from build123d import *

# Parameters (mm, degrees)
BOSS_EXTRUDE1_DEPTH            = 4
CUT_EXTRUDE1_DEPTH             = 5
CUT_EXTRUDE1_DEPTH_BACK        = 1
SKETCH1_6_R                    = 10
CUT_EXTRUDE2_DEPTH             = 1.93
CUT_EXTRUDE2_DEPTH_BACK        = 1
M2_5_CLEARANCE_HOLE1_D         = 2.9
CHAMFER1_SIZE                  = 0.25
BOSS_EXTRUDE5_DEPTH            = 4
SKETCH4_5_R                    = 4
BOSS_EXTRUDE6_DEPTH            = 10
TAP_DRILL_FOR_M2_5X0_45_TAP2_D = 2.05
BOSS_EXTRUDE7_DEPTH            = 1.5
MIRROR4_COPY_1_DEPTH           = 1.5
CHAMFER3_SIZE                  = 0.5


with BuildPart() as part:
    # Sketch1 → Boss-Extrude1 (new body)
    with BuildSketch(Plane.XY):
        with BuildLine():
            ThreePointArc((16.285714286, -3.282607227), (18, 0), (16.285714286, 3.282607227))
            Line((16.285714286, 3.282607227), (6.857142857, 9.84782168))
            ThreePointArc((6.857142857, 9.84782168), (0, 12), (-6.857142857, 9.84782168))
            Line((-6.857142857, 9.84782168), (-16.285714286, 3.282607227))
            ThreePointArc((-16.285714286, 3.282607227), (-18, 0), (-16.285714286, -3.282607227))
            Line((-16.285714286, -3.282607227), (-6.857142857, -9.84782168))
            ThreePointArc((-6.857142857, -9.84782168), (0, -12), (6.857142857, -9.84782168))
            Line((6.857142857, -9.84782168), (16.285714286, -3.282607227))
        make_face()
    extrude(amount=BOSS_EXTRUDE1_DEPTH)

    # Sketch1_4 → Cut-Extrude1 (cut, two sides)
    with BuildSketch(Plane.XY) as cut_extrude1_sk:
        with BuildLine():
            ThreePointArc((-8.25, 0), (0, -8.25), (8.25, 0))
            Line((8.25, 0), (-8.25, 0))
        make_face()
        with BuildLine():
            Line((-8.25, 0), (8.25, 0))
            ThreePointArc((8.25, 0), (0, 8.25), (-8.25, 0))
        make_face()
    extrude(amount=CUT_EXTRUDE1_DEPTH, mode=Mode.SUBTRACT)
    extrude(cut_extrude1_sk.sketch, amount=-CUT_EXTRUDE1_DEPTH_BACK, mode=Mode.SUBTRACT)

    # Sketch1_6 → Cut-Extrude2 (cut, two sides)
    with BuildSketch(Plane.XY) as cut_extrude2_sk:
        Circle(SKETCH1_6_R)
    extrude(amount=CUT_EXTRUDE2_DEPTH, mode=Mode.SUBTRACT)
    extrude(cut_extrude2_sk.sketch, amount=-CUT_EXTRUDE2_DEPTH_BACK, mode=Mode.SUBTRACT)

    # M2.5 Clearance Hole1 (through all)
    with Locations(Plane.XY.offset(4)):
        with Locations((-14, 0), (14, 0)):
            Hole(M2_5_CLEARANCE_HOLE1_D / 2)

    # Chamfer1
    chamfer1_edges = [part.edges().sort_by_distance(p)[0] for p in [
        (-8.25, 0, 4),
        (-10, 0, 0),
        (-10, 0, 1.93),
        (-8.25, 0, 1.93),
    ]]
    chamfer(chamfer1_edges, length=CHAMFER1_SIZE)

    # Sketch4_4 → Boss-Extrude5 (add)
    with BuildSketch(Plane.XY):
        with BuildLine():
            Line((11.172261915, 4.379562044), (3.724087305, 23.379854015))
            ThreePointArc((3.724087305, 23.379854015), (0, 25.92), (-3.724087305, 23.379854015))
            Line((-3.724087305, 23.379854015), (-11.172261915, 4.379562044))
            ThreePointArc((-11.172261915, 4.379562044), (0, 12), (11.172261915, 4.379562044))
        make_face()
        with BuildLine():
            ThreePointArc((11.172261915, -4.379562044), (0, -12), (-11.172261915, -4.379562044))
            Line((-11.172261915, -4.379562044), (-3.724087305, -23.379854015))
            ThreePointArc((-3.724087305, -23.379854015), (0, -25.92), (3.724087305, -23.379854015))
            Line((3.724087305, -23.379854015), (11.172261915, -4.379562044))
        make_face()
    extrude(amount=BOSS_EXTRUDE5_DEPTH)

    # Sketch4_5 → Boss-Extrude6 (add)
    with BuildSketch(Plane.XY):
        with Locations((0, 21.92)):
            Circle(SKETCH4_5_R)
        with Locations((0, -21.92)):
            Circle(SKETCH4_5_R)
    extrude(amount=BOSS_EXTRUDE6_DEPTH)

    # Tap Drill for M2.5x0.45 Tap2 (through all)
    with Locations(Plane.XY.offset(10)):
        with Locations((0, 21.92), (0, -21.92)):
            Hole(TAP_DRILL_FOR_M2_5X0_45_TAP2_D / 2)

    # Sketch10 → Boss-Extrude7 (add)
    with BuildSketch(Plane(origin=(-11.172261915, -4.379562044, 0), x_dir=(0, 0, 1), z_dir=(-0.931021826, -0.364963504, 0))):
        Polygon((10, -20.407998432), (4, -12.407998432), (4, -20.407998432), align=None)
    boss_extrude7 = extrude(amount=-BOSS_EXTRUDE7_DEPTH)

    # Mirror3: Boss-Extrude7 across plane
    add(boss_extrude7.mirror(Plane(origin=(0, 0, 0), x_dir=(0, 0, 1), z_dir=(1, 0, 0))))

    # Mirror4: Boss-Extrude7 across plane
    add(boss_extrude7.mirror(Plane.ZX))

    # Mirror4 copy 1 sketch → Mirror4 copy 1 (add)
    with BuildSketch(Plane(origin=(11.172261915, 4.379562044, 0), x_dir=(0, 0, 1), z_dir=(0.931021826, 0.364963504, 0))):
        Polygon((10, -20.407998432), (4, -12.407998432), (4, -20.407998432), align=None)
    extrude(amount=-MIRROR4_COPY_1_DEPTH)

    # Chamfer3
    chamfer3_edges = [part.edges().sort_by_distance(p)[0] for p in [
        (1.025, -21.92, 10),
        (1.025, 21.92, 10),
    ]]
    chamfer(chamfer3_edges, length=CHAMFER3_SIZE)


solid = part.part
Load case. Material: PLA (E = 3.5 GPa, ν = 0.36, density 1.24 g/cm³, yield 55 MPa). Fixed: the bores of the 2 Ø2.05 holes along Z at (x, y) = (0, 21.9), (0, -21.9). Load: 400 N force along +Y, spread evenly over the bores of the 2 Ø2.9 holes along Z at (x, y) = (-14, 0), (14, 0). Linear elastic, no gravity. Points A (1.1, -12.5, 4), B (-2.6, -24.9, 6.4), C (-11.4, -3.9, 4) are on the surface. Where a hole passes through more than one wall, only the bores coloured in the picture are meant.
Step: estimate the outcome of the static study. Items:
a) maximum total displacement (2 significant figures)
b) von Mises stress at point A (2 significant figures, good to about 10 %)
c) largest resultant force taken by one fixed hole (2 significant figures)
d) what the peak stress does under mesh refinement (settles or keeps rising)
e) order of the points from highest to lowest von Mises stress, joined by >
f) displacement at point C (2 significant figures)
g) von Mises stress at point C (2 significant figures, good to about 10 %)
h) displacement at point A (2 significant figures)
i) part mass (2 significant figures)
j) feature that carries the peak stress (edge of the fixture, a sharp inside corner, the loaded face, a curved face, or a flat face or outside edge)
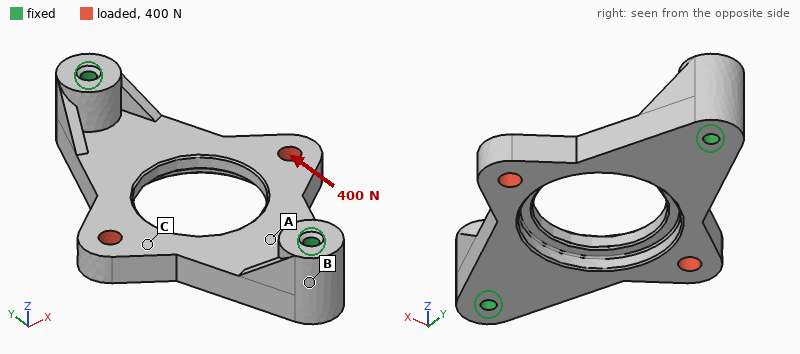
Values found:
65 µm
3.0 MPa
200 N
keeps rising
C > A > B
40 µm
5.5 MPa
12 µm
3.9 g
edge of the fixture
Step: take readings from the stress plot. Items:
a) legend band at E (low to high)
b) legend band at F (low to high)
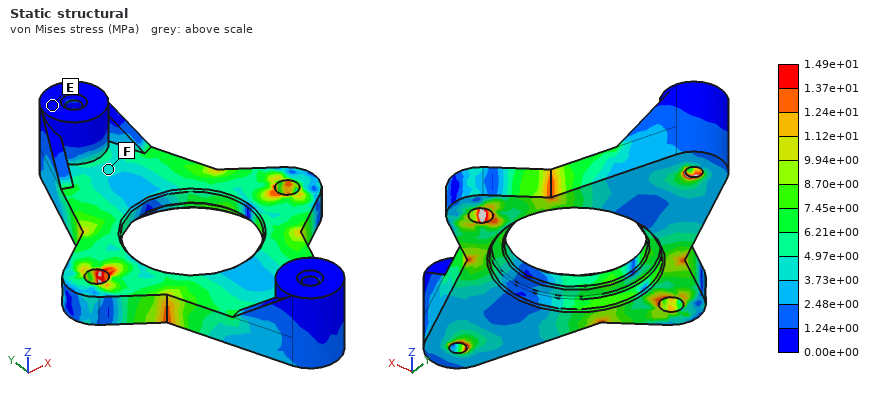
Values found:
0.00e+00 to 1.24e+00 MPa
3.73e+00 to 4.97e+00 MPa
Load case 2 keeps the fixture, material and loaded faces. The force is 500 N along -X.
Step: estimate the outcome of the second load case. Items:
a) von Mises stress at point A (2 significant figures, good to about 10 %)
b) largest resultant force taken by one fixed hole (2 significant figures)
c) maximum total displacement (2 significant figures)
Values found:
7.2 MPa
250 N
0.15 mm
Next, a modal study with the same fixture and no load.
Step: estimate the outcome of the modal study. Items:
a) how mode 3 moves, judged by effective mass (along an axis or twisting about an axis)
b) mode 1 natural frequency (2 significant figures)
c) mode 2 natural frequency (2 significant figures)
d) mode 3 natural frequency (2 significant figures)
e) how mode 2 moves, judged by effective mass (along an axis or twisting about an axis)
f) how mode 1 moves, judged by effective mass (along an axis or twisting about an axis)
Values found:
along X
2700 Hz
2800 Hz
7100 Hz
along Z
twisting about Y
